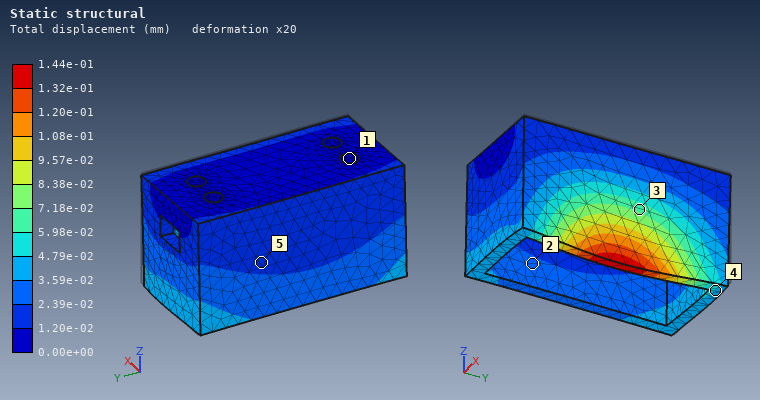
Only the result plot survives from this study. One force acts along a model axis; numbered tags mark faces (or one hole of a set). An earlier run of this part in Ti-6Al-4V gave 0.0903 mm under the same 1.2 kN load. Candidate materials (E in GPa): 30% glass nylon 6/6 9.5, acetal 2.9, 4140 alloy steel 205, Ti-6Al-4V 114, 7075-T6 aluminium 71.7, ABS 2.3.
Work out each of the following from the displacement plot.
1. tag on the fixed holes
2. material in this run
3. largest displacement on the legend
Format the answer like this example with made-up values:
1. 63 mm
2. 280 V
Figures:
1. 1
2. 7075-T6 aluminium
3. 1.44e-01 mm
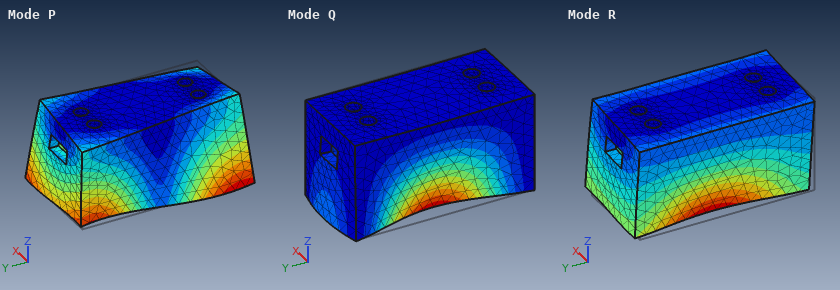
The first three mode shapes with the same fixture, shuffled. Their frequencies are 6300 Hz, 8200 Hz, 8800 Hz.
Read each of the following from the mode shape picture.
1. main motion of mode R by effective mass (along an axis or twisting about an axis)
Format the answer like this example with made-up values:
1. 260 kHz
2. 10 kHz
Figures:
1. along X
